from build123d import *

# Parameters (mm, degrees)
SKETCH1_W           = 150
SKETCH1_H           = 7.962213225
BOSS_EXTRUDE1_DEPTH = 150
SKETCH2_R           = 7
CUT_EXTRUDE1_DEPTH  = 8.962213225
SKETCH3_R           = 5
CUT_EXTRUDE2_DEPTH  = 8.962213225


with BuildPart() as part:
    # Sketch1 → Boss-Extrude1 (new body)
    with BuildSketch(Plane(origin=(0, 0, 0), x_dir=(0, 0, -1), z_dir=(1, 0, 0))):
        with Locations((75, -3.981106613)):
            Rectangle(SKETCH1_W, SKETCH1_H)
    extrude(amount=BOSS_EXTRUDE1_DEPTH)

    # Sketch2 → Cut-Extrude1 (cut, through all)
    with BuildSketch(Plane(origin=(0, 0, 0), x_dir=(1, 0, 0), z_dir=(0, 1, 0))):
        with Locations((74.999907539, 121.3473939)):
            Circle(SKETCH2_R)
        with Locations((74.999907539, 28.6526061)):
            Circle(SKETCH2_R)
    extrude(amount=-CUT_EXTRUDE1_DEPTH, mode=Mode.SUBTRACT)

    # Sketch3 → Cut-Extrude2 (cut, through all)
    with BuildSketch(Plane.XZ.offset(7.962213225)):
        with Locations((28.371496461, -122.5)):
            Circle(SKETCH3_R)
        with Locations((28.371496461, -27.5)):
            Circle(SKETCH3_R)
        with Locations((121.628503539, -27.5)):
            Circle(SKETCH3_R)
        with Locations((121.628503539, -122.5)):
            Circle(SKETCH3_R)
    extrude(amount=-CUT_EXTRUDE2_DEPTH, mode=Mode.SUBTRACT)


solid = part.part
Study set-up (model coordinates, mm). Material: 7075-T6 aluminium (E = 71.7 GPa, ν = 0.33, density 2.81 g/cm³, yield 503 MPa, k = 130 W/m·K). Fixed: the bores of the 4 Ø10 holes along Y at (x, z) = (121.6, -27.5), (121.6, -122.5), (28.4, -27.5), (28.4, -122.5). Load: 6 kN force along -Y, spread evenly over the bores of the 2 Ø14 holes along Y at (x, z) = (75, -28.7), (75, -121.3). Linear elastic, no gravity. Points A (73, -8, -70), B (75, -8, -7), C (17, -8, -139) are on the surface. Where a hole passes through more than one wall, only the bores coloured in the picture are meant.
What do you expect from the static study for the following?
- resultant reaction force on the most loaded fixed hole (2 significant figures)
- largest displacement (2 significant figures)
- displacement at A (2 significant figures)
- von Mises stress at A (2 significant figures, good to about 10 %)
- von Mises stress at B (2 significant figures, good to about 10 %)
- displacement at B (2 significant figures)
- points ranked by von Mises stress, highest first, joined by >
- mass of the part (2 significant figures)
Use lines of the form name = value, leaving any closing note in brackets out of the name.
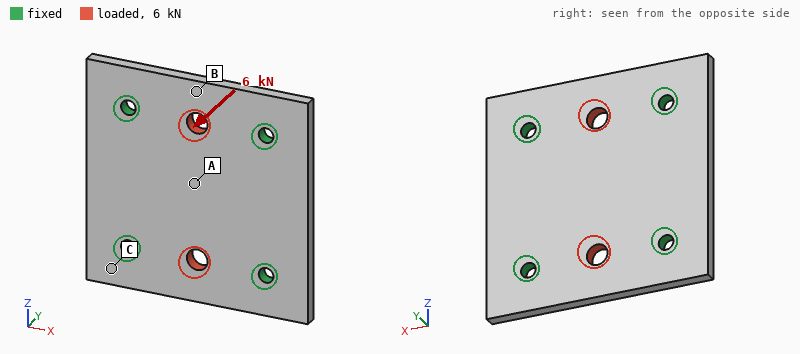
resultant reaction force on the most loaded fixed hole = 1.5 kN
largest displacement = 94 µm
displacement at A = 57 µm
von Mises stress at A = 22 MPa
von Mises stress at B = 45 MPa
displacement at B = 76 µm
points ranked by von Mises stress, highest first, joined by > = B > A > C
mass of the part = 490 g
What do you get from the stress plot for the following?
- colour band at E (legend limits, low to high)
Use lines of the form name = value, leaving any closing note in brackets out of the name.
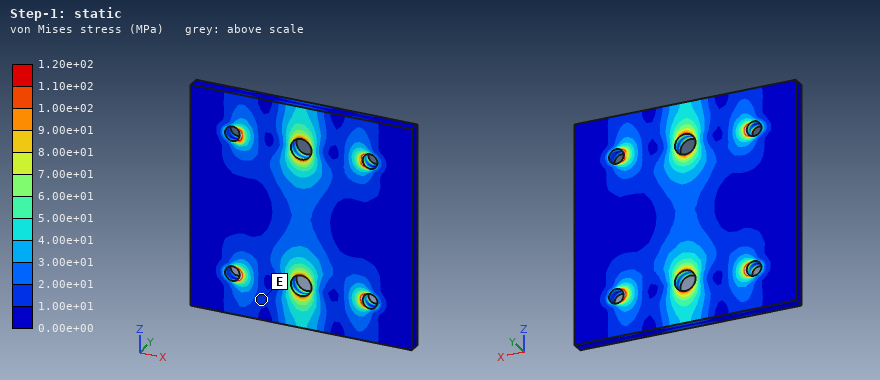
colour band at E = 1.00e+01 to 2.00e+01 MPa
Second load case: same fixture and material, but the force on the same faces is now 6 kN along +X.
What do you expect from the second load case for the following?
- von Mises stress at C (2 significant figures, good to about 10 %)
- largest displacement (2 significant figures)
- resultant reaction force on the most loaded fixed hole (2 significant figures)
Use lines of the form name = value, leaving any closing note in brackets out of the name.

von Mises stress at C = 1.5 MPa
largest displacement = 3.7 µm
resultant reaction force on the most loaded fixed hole = 1.5 kN
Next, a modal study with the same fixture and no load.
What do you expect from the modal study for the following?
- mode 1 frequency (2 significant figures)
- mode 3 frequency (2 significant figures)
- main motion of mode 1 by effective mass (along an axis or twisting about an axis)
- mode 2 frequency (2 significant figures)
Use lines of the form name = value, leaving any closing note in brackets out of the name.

mode 1 frequency = 3400 Hz
mode 3 frequency = 4300 Hz
main motion of mode 1 by effective mass = along Y
mode 2 frequency = 4200 Hz
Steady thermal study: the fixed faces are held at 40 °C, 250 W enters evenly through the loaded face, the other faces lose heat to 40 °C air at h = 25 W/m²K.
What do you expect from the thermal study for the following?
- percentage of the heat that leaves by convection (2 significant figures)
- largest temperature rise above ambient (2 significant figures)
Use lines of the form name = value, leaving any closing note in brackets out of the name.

percentage of the heat that leaves by convection = 8.6 %
largest temperature rise above ambient = 56 K
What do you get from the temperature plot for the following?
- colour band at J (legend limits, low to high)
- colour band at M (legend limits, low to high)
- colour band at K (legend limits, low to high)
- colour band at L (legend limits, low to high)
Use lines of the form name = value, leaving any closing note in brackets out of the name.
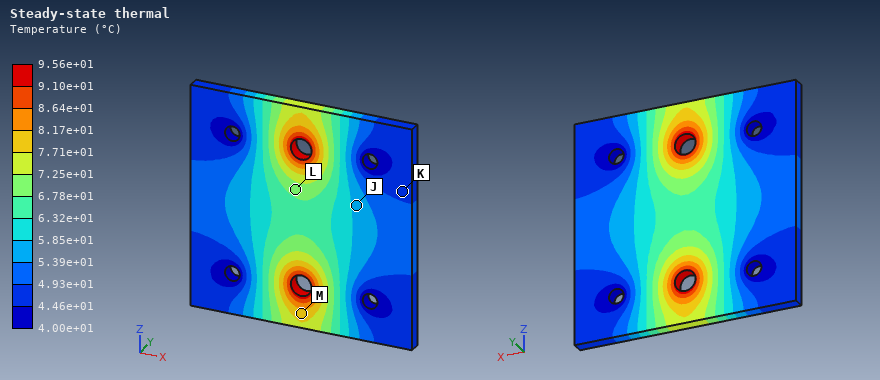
colour band at J = 5.39e+01 to 5.85e+01 °C
colour band at M = 7.71e+01 to 8.17e+01 °C
colour band at K = 4.46e+01 to 4.93e+01 °C
colour band at L = 6.78e+01 to 7.25e+01 °C
